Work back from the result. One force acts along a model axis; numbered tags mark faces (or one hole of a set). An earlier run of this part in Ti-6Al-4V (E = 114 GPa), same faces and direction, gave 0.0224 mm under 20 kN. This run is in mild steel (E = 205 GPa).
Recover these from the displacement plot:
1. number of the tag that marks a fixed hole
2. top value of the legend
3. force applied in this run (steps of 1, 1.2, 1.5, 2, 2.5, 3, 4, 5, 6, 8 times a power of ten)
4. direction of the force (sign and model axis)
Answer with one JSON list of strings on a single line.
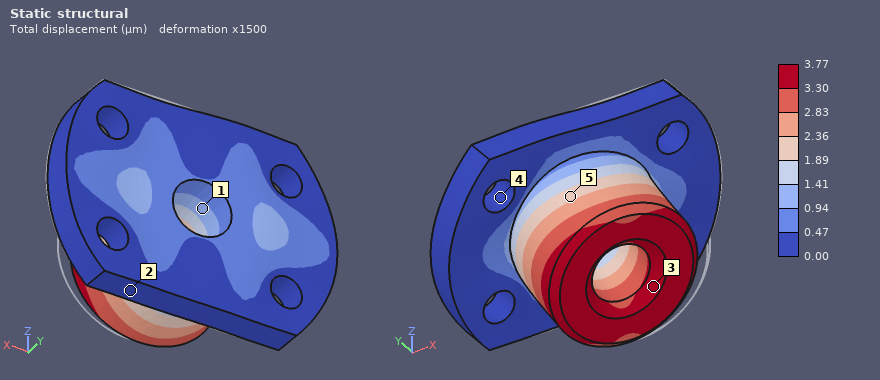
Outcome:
["4", "3.77 µm", "6 kN", "-X"]
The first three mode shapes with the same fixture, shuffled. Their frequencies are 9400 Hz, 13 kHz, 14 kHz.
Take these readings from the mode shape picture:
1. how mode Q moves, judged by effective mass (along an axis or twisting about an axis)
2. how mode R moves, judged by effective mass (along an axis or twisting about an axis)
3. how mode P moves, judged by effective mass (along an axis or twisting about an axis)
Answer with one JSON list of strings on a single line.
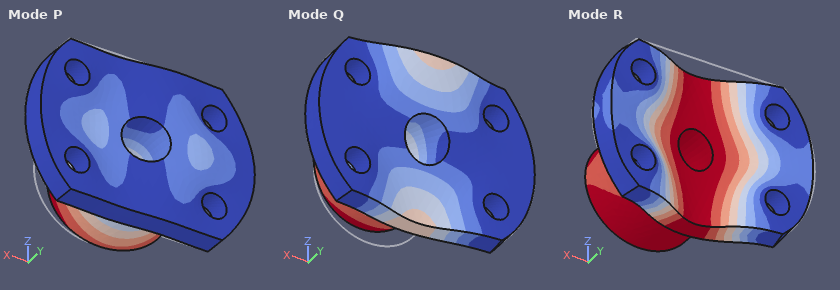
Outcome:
["along Z", "along Y", "along X"]
